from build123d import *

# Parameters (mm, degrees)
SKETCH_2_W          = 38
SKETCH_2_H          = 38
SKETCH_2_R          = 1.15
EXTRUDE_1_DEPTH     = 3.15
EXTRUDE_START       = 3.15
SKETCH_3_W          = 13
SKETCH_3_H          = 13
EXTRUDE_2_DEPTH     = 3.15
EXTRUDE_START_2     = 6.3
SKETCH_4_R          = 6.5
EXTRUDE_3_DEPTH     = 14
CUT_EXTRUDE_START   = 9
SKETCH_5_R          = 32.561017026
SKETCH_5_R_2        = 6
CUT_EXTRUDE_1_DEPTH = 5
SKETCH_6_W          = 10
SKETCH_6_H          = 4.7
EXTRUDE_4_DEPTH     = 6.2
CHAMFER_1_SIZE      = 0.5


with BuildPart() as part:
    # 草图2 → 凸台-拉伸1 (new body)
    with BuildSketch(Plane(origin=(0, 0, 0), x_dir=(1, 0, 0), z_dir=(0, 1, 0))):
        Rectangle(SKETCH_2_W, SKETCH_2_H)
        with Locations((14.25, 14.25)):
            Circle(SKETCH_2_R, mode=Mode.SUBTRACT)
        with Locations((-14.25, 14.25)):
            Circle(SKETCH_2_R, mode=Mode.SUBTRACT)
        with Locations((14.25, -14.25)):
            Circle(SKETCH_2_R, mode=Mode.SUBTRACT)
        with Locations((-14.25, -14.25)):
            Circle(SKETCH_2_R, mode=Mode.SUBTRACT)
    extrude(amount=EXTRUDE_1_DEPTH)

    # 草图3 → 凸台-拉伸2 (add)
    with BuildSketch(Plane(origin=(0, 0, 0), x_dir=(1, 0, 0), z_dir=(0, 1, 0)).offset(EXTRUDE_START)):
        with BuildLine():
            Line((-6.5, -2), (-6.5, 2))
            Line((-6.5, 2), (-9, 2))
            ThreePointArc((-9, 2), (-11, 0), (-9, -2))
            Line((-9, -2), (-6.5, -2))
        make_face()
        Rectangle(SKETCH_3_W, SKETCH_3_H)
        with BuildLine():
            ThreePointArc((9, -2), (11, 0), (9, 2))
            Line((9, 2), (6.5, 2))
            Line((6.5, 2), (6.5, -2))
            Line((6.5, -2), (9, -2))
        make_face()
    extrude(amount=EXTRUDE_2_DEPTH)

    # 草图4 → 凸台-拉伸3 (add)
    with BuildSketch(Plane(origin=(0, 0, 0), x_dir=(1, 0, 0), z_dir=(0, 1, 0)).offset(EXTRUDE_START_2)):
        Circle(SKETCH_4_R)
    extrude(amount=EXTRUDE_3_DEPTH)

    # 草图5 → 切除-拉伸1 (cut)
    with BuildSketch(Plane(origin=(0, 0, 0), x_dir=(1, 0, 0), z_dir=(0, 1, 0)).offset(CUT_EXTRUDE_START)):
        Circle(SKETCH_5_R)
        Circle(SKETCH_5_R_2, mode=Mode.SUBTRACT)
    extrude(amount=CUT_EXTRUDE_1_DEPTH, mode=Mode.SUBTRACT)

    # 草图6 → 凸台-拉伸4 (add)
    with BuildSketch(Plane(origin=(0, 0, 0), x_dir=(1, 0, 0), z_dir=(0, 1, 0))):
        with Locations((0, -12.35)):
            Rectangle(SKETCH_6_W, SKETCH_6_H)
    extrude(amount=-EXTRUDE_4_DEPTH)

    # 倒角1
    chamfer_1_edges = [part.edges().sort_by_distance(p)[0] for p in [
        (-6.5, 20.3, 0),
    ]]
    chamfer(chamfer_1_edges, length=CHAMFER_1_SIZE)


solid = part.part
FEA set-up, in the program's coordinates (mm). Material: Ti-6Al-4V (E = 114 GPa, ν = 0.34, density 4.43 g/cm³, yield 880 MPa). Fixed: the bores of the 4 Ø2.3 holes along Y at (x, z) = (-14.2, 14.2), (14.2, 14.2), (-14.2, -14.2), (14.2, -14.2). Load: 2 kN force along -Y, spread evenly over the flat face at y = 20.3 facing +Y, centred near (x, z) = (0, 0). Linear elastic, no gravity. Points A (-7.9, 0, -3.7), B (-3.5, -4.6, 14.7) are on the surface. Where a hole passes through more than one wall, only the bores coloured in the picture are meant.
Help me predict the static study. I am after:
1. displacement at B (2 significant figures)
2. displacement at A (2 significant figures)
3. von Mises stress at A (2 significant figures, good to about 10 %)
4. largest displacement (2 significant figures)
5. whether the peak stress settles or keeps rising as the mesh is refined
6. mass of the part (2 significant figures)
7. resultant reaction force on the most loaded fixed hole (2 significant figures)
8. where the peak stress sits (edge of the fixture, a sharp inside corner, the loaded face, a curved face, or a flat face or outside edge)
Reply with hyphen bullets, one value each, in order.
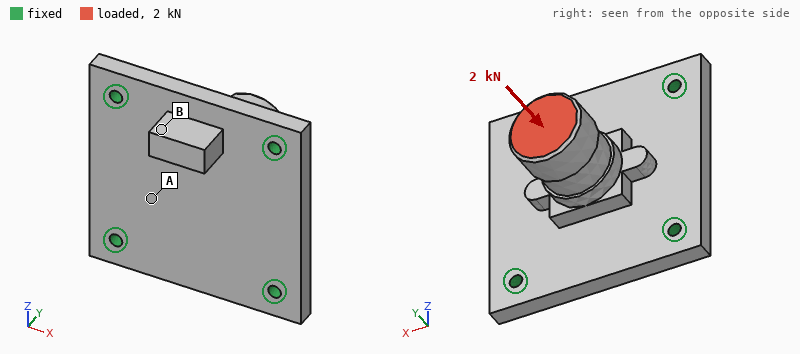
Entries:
- 17 µm
- 26 µm
- 67 MPa
- 31 µm
- keeps rising
- 32 g
- 520 N
- edge of the fixture
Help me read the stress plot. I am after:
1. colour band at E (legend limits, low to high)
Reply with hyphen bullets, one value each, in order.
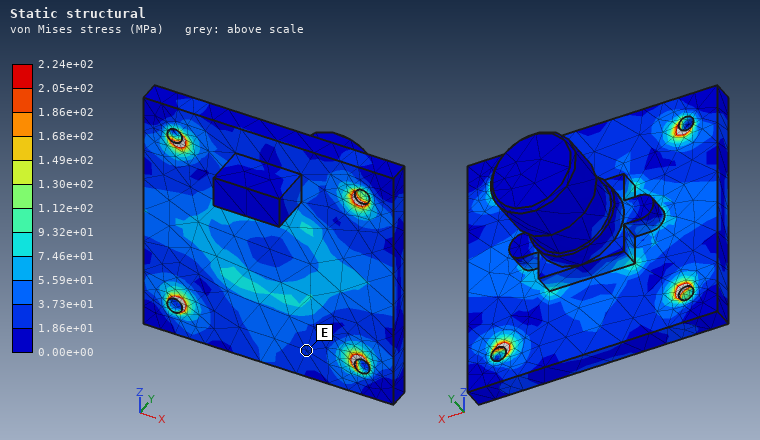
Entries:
- 1.86e+01 to 3.73e+01 MPa
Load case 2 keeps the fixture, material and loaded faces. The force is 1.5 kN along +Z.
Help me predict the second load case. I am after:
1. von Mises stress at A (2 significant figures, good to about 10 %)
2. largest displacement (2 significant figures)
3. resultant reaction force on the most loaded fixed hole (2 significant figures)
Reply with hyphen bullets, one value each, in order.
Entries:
- 92 MPa
- 92 µm
- 720 N
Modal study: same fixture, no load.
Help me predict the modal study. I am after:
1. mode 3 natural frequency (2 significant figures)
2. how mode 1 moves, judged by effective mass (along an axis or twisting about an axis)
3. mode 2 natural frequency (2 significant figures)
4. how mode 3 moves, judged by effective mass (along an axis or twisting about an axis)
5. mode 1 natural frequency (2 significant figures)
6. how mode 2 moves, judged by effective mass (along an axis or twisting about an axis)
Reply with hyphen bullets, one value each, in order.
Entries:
- 11 kHz
- along Y
- 10 kHz
- along X
- 9800 Hz
- along Z
